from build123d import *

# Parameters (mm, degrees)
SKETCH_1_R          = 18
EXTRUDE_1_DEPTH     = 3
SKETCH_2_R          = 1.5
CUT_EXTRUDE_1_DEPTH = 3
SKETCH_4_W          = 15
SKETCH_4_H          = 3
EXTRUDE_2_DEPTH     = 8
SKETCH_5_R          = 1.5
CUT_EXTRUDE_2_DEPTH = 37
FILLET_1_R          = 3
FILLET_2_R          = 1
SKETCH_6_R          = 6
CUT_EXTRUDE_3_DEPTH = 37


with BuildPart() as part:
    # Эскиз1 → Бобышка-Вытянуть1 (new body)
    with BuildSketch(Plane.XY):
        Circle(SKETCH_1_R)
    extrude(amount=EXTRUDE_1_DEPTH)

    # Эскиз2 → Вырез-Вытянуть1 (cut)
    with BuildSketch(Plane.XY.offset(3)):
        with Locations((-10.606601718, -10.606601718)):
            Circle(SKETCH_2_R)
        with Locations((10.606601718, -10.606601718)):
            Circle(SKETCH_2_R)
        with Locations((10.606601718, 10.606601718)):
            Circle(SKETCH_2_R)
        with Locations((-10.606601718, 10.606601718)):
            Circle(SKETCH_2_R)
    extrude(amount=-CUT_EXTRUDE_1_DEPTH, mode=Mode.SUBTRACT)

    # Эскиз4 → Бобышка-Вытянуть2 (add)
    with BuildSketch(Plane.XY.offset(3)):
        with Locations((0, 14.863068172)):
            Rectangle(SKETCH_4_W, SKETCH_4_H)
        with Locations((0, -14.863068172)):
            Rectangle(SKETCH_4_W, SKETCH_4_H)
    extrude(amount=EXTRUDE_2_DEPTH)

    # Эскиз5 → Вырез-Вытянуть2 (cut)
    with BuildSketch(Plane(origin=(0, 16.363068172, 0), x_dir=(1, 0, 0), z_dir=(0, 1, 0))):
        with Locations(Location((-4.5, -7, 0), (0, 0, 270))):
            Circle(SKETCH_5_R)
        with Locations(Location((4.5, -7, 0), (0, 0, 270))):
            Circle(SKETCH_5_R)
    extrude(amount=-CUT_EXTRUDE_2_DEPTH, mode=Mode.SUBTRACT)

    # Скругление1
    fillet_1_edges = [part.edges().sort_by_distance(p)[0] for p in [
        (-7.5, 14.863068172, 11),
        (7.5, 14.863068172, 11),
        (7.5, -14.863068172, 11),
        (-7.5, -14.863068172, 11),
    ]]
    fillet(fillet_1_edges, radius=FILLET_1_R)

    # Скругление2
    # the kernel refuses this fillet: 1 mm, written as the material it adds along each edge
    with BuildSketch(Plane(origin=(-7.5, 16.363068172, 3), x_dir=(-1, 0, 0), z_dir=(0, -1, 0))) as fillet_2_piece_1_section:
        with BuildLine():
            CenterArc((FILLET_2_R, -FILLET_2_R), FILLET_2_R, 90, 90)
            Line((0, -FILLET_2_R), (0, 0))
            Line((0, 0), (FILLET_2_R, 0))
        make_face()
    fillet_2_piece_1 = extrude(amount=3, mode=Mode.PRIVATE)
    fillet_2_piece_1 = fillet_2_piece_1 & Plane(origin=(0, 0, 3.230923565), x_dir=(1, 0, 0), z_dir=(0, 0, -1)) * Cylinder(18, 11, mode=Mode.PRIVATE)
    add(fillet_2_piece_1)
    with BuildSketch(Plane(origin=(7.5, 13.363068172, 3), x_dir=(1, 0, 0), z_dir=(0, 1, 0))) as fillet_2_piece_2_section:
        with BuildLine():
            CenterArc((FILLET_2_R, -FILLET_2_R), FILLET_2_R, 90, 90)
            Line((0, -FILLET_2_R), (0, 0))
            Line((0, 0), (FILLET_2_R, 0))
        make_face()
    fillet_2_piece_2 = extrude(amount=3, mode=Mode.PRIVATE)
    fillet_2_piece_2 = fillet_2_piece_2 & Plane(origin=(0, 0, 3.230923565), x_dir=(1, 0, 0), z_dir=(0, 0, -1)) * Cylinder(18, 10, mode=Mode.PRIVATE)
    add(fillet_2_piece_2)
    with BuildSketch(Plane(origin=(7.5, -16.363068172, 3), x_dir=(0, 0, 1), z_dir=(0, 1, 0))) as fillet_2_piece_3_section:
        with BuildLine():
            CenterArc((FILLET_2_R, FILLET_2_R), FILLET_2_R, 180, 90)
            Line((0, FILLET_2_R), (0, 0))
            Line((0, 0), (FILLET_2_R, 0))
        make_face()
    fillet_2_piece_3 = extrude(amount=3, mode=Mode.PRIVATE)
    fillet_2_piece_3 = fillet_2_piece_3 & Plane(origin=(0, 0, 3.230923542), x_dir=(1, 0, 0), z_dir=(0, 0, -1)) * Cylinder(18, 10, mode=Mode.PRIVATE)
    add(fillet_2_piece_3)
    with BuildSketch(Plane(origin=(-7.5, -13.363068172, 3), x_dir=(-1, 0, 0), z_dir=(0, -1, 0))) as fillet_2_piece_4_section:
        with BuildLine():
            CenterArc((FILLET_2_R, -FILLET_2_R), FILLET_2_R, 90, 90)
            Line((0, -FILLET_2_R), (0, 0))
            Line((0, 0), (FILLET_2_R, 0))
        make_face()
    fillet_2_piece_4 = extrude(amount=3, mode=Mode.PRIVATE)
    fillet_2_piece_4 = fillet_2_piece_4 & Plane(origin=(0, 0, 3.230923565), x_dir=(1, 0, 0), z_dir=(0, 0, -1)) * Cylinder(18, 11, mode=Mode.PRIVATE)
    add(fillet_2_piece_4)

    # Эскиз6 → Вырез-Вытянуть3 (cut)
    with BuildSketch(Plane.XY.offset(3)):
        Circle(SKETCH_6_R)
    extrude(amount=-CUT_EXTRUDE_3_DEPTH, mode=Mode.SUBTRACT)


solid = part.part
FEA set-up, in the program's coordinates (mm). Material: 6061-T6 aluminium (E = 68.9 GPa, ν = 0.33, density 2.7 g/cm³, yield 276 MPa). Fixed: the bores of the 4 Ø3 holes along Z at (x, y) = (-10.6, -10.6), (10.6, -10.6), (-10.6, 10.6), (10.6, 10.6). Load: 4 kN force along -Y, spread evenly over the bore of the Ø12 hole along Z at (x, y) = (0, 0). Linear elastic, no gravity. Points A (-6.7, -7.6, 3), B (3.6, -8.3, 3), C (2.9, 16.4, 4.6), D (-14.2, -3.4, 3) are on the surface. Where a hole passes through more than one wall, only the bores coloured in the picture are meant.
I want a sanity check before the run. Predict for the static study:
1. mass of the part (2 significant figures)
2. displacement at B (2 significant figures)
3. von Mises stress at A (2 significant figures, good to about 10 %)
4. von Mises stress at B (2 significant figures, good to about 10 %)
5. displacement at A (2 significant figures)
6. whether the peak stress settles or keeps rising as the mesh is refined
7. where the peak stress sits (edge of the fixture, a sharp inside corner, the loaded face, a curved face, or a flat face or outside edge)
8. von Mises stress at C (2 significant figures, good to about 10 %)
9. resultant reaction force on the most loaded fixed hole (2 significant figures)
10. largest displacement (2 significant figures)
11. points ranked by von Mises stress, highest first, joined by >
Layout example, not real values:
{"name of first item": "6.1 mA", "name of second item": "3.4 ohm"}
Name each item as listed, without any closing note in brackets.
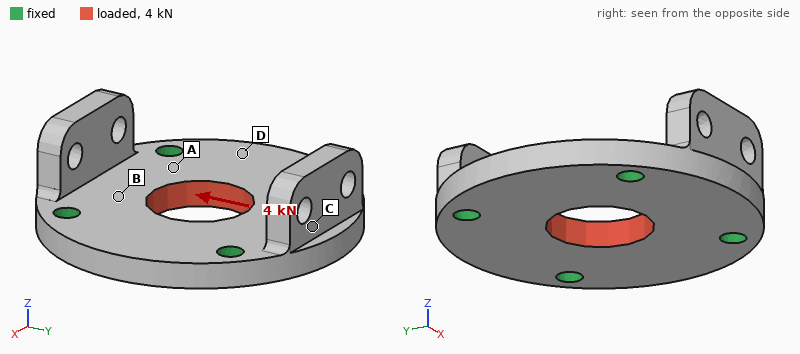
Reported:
{"mass of the part": "8.8 g", "displacement at B": "6.3 µm", "von Mises stress at A": "41 MPa", "von Mises stress at B": "31 MPa", "displacement at A": "3.8 µm", "whether the peak stress settles or keeps rising as the mesh is refined": "keeps rising", "where the peak stress sits": "edge of the fixture", "von Mises stress at C": "15 MPa", "resultant reaction force on the most loaded fixed hole": "1.0 kN", "largest displacement": "8.7 µm", "points ranked by von Mises stress, highest first, joined by >": "A > B > C > D"}
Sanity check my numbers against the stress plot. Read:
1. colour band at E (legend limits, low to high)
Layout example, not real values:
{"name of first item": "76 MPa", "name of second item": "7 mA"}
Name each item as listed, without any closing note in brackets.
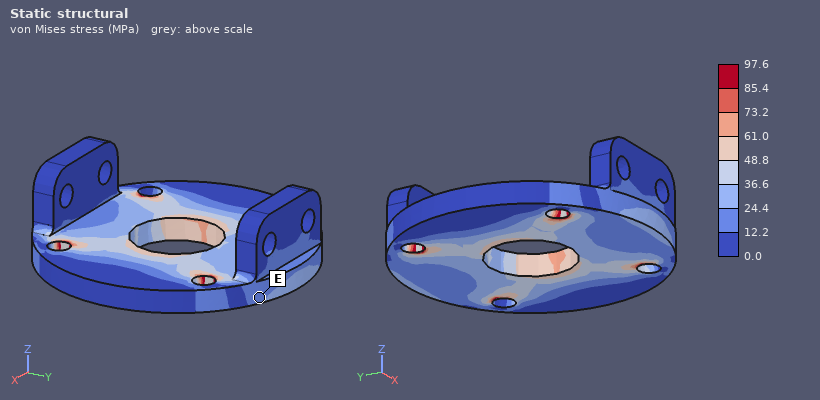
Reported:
{"colour band at E": "12.2 to 24.4 MPa"}
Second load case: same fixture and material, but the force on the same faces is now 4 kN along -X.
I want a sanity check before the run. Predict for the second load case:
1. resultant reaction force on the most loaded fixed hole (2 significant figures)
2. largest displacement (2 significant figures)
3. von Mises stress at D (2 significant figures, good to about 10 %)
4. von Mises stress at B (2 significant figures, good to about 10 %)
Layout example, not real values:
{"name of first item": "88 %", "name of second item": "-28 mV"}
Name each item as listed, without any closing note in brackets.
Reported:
{"resultant reaction force on the most loaded fixed hole": "1.0 kN", "largest displacement": "8.9 µm", "von Mises stress at D": "20 MPa", "von Mises stress at B": "37 MPa"}
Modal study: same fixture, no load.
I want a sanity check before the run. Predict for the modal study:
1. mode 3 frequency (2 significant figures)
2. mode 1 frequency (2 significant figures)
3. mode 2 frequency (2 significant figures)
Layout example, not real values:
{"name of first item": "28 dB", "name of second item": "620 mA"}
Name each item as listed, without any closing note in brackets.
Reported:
{"mode 3 frequency": "28 kHz", "mode 1 frequency": "16 kHz", "mode 2 frequency": "17 kHz"}
